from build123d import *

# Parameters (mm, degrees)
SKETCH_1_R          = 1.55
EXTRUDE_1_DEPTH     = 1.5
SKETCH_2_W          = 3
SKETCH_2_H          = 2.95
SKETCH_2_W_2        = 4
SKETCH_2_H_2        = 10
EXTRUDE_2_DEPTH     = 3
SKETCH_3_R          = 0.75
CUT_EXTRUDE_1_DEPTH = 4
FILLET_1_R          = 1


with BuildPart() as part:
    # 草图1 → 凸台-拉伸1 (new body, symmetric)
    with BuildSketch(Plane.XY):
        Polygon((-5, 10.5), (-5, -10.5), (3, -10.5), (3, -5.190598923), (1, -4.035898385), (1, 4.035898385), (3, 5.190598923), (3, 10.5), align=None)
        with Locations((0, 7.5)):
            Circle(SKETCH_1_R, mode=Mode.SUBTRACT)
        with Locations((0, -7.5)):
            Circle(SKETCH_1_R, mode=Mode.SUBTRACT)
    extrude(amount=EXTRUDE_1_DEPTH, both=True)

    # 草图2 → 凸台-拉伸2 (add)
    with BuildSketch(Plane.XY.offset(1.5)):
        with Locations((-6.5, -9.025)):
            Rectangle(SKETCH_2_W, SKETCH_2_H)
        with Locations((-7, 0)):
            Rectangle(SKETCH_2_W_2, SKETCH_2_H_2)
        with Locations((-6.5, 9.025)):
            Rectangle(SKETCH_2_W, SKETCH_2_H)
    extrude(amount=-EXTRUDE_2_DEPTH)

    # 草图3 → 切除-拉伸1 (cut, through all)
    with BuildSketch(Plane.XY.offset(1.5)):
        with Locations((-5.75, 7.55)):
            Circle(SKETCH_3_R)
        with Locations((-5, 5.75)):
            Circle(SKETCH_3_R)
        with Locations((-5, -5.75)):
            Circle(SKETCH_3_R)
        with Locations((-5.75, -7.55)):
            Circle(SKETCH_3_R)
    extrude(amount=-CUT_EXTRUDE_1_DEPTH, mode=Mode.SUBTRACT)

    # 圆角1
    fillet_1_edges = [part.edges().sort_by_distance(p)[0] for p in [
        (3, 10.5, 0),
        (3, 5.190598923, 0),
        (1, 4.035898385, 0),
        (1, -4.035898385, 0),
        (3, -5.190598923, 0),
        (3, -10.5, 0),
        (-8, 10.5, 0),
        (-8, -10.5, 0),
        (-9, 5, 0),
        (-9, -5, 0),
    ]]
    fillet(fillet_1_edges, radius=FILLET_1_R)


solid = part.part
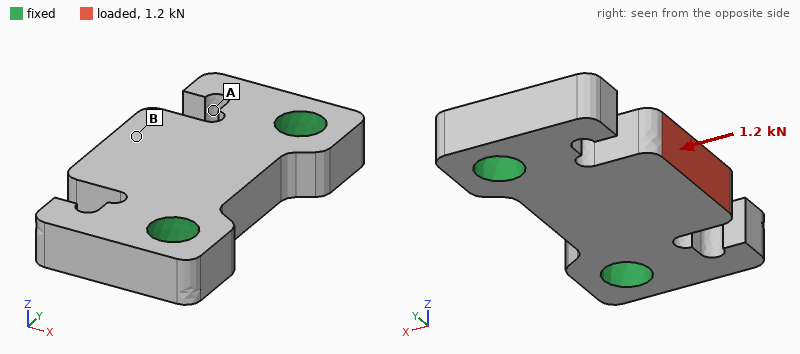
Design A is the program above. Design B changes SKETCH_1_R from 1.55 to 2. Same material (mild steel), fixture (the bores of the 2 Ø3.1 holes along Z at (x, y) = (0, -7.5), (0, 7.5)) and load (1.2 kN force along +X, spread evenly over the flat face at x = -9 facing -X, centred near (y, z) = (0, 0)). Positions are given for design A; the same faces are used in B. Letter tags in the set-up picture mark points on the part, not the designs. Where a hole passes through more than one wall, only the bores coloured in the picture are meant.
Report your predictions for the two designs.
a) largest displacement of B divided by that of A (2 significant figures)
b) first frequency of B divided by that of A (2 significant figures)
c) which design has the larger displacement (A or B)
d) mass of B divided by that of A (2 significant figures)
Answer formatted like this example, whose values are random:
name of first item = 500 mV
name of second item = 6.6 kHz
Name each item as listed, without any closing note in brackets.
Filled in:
largest displacement of B divided by that of A = 0.91
first frequency of B divided by that of A = 1.1
which design has the larger displacement = A
mass of B divided by that of A = 0.95
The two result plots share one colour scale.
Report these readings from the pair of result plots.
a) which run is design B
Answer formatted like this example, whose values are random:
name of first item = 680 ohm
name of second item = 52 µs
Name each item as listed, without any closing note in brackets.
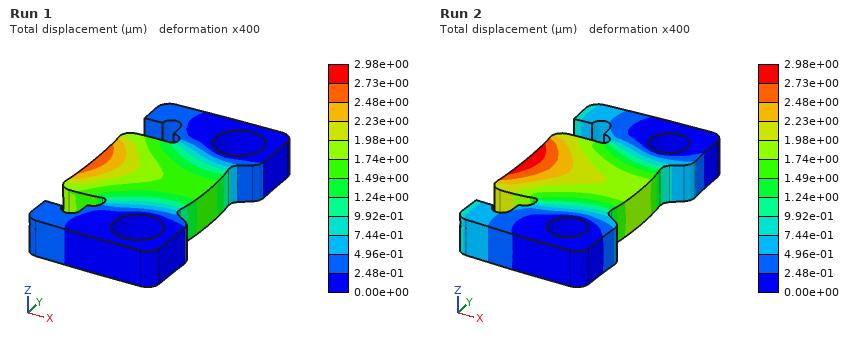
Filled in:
which run is design B = Run 1
